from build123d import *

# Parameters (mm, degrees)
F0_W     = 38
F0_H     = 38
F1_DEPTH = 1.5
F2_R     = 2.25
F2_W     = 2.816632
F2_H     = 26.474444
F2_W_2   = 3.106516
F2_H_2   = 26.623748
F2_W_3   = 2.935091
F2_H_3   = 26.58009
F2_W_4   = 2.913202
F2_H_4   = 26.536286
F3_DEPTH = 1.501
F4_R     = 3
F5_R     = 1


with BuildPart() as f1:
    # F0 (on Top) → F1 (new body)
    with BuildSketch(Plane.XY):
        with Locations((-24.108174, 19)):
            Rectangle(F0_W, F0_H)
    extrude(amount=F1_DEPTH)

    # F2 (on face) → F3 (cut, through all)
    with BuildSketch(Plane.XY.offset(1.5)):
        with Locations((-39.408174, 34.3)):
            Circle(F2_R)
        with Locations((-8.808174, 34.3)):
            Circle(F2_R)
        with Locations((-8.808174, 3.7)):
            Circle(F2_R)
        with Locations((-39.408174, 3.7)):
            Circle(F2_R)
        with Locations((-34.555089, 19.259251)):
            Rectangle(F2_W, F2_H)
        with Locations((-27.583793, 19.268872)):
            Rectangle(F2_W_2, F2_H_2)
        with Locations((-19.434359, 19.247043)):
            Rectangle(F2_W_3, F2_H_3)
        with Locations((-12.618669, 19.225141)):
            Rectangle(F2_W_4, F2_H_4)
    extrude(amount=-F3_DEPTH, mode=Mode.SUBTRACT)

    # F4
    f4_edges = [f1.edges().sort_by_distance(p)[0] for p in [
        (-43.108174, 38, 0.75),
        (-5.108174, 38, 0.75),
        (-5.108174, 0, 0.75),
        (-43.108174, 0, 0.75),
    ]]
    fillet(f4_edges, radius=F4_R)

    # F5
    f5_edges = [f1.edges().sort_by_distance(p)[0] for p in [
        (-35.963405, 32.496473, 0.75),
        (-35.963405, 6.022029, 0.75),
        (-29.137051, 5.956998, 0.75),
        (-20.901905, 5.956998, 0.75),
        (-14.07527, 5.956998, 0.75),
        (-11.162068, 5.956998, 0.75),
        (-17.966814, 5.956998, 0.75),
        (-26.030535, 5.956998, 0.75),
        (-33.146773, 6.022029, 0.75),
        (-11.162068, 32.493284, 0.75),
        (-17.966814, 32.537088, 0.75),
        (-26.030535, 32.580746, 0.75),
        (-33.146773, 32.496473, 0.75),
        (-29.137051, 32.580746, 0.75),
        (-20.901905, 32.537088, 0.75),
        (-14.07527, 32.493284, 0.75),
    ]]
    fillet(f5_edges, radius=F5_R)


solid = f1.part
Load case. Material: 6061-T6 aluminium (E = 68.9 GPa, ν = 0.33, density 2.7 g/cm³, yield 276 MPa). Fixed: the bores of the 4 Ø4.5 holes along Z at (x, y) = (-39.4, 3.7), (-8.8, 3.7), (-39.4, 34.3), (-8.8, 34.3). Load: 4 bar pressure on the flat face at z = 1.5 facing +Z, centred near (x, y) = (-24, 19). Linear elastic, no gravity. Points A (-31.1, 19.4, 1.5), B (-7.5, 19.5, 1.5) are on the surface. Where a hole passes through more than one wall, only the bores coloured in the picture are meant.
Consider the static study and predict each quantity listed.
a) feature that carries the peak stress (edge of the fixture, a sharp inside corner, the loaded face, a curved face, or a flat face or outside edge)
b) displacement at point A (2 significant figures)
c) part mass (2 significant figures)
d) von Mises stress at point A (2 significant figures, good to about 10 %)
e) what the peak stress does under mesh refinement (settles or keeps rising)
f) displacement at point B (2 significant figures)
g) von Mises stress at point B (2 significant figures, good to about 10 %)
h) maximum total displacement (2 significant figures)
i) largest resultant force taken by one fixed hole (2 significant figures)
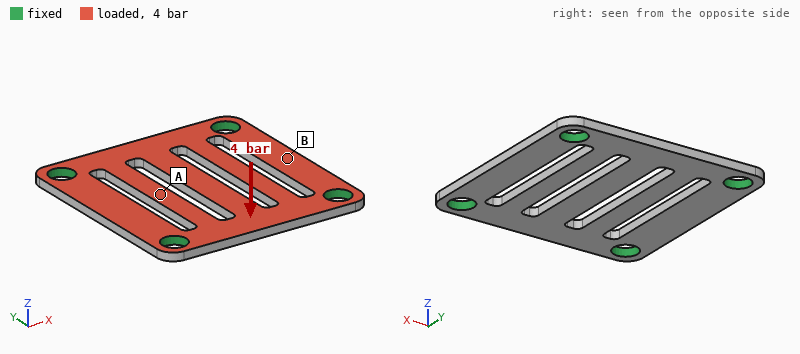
edge of the fixture
0.11 mm
4.3 g
55 MPa
keeps rising
0.027 mm
30 MPa
0.17 mm
110 N
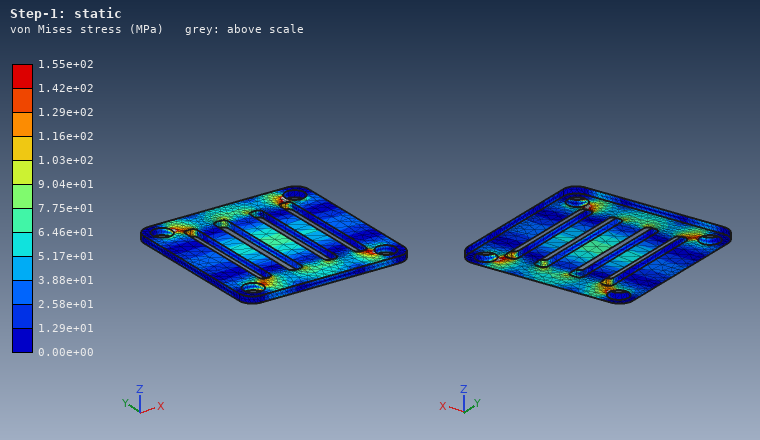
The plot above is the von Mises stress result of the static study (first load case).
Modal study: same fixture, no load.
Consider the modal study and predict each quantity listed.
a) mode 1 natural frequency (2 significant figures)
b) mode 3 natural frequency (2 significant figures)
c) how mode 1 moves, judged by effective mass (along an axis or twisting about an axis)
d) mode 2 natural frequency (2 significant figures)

4800 Hz
8000 Hz
along Z
7400 Hz
